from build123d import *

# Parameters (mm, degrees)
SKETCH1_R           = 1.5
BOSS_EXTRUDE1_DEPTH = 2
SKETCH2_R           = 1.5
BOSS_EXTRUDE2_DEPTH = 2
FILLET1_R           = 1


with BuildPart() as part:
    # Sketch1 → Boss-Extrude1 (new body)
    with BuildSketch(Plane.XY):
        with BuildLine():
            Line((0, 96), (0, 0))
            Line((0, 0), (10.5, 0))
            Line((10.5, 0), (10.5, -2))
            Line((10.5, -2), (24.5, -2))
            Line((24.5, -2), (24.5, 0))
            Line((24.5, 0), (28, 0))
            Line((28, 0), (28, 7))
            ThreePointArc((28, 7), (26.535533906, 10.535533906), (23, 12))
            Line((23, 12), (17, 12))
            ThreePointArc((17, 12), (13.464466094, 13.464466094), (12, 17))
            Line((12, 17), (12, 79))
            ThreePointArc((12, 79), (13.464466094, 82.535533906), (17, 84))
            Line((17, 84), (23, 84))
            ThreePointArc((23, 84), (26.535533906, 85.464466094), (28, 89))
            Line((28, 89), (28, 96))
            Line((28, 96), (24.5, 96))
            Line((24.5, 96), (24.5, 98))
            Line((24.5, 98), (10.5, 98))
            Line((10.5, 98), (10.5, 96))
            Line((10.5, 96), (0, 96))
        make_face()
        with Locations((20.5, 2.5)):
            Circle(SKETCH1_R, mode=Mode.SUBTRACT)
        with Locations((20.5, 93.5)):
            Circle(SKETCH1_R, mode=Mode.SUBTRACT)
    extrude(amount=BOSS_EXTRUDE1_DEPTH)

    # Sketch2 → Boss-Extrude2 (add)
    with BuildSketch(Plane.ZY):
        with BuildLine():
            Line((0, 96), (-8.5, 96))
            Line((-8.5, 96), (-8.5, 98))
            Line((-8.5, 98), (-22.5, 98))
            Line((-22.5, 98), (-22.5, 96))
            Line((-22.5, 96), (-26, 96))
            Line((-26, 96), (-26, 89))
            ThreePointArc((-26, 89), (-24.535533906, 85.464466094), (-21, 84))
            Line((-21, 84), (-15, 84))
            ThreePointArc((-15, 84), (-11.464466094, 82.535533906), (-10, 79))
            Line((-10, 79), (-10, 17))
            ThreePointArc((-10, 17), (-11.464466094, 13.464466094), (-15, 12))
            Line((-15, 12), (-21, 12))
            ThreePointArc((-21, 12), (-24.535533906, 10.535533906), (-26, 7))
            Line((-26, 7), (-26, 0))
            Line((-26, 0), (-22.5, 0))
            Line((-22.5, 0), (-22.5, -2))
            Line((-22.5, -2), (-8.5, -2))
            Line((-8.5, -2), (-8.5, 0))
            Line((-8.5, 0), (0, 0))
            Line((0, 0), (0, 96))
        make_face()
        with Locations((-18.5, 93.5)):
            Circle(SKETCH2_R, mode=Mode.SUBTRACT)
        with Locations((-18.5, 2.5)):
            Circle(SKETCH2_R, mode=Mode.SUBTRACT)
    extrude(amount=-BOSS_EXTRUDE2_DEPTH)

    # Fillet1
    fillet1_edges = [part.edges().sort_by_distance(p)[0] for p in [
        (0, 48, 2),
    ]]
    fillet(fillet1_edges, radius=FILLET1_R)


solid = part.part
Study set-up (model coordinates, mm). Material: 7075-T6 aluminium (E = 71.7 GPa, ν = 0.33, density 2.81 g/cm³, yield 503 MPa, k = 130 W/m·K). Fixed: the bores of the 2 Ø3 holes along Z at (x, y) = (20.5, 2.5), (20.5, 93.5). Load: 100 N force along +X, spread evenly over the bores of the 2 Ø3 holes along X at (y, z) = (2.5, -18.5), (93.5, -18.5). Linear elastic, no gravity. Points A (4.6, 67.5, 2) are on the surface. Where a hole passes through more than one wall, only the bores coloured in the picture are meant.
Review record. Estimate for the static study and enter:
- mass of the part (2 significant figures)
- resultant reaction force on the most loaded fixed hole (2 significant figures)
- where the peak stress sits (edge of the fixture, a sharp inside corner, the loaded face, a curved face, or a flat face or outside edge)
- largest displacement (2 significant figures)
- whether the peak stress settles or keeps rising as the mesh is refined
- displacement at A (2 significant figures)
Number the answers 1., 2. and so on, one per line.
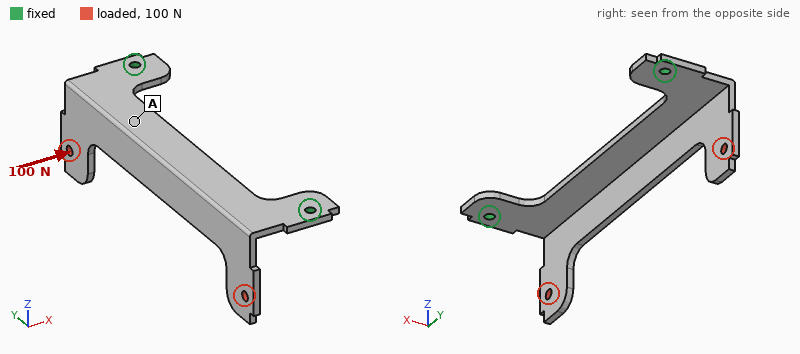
1. 17 g
2. 50 N
3. edge of the fixture
4. 0.92 mm
5. keeps rising
6. 0.18 mm
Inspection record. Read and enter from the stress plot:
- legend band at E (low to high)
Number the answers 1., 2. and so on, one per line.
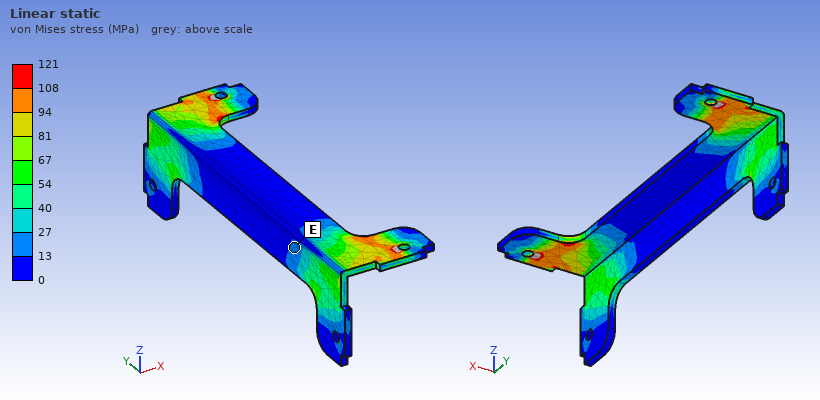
1. 13 to 27 MPa
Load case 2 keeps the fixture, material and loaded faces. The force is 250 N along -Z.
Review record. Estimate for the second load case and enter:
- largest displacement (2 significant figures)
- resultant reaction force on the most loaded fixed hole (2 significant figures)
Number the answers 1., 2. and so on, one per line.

1. 1.00 mm
2. 130 N
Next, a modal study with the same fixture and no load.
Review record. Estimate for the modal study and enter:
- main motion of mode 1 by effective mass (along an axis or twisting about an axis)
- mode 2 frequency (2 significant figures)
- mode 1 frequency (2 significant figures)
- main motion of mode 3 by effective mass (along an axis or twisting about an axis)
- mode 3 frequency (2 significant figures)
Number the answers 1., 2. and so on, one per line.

1. along Z
2. 1400 Hz
3. 890 Hz
4. along Z
5. 2300 Hz
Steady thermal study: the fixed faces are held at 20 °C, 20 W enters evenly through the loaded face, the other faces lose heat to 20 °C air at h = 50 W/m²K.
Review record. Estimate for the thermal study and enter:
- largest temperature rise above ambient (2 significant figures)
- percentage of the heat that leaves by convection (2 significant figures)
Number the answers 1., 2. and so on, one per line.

1. 76 K
2. 47 %
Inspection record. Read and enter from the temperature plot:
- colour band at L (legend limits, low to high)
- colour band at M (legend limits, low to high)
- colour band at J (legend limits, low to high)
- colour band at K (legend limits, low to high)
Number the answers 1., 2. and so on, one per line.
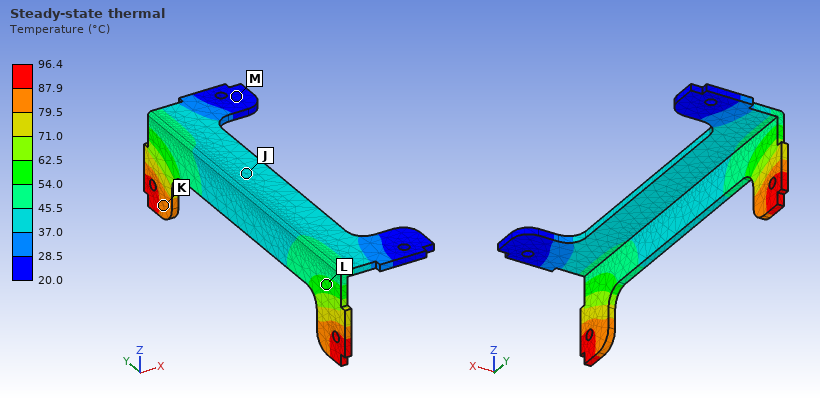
1. 54.0 to 62.5 °C
2. 20.0 to 28.5 °C
3. 37.0 to 45.5 °C
4. 79.5 to 87.9 °C
